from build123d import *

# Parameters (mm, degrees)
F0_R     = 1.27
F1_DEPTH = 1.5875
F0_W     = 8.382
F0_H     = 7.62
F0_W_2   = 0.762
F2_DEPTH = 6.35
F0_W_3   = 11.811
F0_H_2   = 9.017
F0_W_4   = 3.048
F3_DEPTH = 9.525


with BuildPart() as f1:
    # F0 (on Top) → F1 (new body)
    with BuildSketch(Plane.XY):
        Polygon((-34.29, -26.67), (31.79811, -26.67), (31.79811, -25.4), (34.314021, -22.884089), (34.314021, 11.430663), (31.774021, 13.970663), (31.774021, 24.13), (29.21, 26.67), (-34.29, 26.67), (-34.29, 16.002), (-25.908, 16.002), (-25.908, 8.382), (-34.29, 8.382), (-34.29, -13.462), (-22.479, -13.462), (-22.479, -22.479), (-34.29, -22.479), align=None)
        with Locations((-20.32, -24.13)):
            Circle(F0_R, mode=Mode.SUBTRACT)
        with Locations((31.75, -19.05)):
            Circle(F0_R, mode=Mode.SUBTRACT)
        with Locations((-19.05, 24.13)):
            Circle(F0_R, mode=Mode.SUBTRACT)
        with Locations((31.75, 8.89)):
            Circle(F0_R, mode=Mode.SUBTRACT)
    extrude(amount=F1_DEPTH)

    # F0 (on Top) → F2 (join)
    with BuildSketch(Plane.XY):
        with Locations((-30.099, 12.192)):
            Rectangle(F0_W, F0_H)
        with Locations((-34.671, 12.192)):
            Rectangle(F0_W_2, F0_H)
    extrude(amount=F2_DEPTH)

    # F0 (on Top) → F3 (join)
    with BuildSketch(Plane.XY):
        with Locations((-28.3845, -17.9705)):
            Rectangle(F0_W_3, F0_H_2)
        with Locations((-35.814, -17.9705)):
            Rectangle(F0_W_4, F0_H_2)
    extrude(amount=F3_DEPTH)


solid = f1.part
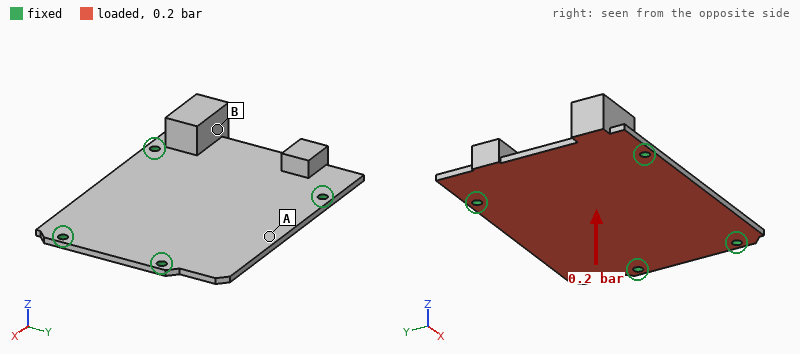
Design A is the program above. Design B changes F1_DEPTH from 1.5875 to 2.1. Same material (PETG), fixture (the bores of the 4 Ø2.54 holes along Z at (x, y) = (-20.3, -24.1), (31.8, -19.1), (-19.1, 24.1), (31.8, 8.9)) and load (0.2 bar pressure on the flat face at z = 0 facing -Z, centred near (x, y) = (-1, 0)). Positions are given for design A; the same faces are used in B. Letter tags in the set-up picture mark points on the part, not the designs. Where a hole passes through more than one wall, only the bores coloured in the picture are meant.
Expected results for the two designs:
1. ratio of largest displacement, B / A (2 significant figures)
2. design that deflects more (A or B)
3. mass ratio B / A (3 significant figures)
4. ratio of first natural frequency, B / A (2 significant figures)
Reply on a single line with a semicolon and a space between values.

0.45; A; 1.25; 1.4
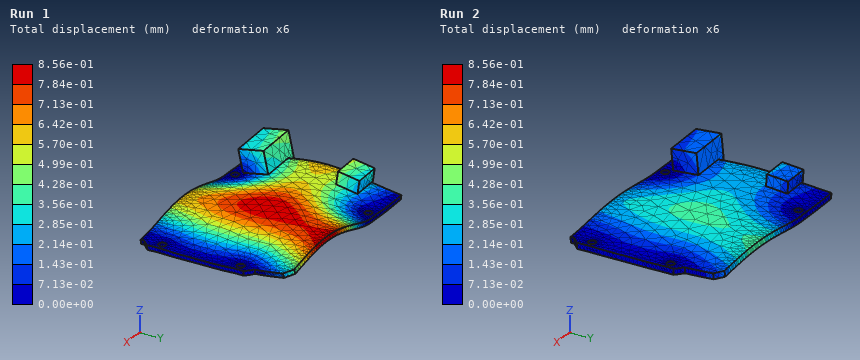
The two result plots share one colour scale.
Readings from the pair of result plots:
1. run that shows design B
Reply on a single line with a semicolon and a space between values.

Run 2
